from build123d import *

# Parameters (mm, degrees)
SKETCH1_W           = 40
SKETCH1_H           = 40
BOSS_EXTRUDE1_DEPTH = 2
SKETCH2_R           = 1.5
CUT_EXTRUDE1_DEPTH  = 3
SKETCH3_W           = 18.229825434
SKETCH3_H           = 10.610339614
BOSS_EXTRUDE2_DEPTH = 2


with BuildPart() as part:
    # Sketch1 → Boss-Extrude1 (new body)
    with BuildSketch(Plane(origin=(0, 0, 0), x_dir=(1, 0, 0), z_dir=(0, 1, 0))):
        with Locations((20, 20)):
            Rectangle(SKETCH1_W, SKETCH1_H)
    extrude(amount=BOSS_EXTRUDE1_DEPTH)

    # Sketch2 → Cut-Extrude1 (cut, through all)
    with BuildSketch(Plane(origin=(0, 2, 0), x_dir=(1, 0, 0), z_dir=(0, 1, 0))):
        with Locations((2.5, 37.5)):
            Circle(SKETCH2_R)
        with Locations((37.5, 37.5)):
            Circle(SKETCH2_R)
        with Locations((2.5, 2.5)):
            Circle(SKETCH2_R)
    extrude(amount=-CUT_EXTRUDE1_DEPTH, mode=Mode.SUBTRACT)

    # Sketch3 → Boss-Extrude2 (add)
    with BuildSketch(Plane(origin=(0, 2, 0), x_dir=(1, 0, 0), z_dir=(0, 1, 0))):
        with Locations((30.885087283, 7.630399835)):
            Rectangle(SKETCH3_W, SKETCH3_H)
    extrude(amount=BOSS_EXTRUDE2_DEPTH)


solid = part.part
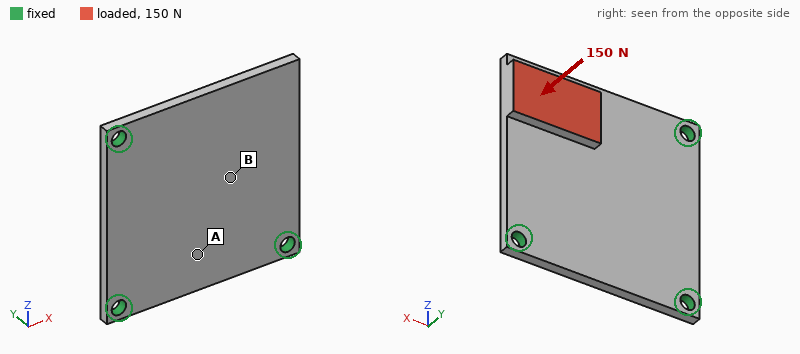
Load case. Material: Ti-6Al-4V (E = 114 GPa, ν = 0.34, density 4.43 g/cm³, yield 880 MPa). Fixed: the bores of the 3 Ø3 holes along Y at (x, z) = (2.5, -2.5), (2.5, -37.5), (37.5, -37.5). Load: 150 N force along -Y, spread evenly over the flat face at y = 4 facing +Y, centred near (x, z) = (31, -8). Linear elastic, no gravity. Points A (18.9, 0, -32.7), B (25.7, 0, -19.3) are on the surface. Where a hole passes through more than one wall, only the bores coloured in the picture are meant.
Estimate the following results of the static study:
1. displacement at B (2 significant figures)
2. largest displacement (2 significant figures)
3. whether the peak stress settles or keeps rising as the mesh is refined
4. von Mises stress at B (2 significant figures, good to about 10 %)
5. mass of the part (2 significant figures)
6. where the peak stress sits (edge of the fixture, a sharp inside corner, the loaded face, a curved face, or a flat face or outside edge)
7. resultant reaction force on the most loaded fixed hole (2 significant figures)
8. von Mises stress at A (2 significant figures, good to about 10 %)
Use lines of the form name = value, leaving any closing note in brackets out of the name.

displacement at B = 0.078 mm
largest displacement = 0.31 mm
whether the peak stress settles or keeps rising as the mesh is refined = keeps rising
von Mises stress at B = 56 MPa
mass of the part = 16 g
where the peak stress sits = edge of the fixture
resultant reaction force on the most loaded fixed hole = 100 N
von Mises stress at A = 28 MPa
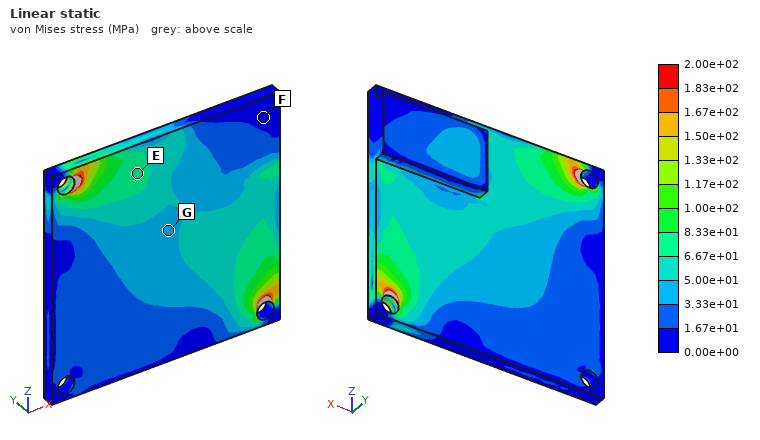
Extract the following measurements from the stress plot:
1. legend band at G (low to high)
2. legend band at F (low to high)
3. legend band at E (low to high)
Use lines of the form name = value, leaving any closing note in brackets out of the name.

legend band at G = 3.33e+01 to 5.00e+01 MPa
legend band at F = 0.00e+00 to 1.67e+01 MPa
legend band at E = 6.67e+01 to 8.33e+01 MPa
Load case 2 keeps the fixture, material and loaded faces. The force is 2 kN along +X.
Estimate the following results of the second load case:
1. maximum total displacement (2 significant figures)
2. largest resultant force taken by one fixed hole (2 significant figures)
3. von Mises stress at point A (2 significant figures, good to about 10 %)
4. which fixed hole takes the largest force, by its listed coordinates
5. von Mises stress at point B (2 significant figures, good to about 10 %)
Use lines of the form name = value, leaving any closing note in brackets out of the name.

maximum total displacement = 0.57 mm
largest resultant force taken by one fixed hole = 1.2 kN
von Mises stress at point A = 49 MPa
which fixed hole takes the largest force, by its listed coordinates = (2.5, -2.5)
von Mises stress at point B = 130 MPa
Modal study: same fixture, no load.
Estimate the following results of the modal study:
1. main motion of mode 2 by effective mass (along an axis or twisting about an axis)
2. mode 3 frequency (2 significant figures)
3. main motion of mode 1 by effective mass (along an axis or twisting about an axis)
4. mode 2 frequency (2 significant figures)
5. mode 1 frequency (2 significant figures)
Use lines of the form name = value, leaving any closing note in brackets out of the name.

main motion of mode 2 by effective mass = along Y
mode 3 frequency = 8200 Hz
main motion of mode 1 by effective mass = along Y
mode 2 frequency = 6100 Hz
mode 1 frequency = 2000 Hz
